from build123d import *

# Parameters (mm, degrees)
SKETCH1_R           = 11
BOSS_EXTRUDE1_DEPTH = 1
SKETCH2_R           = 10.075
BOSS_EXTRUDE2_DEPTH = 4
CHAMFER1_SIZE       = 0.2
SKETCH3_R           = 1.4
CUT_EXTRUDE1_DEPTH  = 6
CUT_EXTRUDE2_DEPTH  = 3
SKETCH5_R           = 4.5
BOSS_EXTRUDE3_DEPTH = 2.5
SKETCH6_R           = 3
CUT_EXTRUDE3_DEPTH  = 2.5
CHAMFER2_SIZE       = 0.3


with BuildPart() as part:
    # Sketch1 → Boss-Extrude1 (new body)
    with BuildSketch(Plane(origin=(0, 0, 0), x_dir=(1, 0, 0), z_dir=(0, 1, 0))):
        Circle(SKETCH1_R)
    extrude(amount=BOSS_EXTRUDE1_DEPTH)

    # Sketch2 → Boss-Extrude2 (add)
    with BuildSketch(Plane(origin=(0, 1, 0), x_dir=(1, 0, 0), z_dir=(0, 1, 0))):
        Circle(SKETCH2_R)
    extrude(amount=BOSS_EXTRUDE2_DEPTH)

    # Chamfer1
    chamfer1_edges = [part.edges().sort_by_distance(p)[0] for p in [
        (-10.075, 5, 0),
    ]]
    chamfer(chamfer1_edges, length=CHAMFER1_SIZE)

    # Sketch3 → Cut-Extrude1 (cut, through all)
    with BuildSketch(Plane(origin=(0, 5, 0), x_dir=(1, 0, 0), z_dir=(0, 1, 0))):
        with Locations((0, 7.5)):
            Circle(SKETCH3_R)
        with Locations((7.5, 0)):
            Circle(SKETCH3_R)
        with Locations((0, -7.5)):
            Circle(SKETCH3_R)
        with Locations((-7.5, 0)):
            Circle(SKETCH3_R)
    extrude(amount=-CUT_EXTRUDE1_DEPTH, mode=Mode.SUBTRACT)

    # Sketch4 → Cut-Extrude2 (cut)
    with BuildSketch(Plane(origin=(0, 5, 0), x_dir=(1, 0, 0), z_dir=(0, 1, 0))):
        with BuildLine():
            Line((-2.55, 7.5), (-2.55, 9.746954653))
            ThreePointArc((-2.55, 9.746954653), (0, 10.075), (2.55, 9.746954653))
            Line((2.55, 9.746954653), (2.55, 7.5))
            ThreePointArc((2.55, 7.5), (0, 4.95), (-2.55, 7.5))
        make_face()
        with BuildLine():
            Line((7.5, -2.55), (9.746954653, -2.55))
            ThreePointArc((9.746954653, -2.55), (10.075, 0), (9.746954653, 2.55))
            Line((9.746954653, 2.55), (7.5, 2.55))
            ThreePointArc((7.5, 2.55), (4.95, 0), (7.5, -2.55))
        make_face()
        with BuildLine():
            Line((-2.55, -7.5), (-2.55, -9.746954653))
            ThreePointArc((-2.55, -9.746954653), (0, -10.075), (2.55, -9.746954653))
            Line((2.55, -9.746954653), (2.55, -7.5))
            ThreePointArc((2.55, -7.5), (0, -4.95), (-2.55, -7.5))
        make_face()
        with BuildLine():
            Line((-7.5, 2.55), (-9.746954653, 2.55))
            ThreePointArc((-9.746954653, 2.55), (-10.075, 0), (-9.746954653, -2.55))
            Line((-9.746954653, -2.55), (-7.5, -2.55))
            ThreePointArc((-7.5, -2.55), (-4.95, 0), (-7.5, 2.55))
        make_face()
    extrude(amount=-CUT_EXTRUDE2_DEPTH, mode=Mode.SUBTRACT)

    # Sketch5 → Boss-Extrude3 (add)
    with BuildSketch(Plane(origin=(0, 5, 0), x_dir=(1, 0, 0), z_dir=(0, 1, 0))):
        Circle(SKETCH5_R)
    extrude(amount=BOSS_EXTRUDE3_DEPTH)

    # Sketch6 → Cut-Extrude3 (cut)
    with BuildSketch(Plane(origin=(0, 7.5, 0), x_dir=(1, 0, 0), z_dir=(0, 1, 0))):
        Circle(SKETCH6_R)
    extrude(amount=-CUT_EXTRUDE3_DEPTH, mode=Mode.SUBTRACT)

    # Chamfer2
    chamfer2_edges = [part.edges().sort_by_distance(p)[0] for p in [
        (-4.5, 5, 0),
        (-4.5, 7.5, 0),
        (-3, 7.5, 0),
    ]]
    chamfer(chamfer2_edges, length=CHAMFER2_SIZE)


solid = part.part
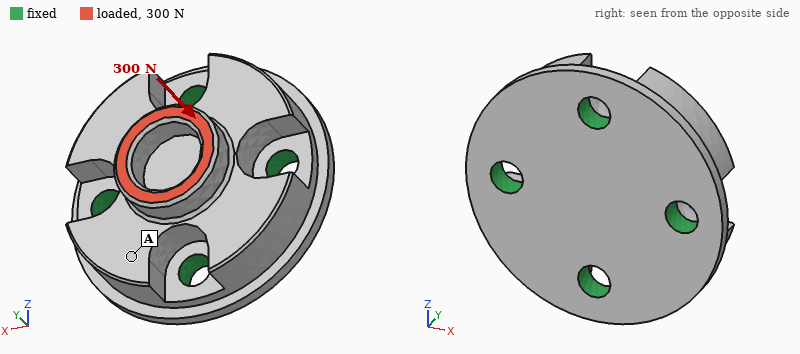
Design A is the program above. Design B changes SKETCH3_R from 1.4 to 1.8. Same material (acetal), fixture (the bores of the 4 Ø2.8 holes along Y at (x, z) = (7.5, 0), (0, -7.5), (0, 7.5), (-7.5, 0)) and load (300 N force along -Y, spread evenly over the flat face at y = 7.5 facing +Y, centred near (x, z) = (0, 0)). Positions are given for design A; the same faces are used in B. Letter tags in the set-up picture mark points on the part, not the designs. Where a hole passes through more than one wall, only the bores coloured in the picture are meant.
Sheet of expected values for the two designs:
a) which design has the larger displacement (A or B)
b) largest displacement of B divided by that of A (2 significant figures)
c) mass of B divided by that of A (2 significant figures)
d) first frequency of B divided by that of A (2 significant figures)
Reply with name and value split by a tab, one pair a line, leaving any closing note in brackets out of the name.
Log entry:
which design has the larger displacement	A
largest displacement of B divided by that of A	0.85
mass of B divided by that of A	0.98
first frequency of B divided by that of A	1.2
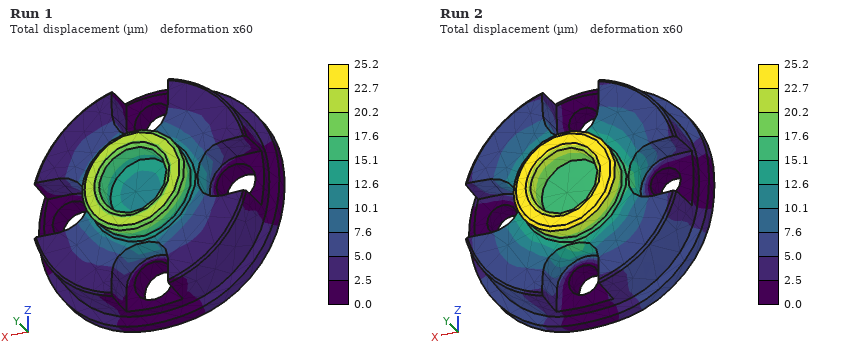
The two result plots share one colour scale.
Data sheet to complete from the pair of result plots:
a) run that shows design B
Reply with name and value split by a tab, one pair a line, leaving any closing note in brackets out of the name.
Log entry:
run that shows design B	Run 1
